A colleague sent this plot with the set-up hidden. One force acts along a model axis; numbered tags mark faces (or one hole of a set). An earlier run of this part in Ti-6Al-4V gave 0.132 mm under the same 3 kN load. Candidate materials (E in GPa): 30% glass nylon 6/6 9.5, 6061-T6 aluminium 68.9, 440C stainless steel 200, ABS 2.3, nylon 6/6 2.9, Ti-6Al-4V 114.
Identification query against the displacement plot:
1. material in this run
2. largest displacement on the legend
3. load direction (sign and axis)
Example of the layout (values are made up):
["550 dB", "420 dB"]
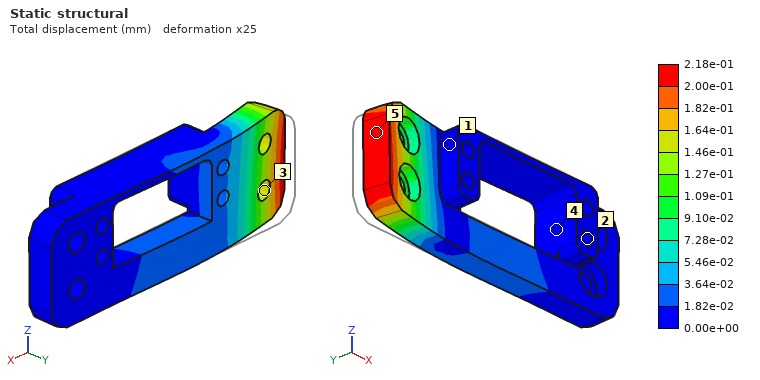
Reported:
["6061-T6 aluminium", "2.18e-01 mm", "-Y"]
